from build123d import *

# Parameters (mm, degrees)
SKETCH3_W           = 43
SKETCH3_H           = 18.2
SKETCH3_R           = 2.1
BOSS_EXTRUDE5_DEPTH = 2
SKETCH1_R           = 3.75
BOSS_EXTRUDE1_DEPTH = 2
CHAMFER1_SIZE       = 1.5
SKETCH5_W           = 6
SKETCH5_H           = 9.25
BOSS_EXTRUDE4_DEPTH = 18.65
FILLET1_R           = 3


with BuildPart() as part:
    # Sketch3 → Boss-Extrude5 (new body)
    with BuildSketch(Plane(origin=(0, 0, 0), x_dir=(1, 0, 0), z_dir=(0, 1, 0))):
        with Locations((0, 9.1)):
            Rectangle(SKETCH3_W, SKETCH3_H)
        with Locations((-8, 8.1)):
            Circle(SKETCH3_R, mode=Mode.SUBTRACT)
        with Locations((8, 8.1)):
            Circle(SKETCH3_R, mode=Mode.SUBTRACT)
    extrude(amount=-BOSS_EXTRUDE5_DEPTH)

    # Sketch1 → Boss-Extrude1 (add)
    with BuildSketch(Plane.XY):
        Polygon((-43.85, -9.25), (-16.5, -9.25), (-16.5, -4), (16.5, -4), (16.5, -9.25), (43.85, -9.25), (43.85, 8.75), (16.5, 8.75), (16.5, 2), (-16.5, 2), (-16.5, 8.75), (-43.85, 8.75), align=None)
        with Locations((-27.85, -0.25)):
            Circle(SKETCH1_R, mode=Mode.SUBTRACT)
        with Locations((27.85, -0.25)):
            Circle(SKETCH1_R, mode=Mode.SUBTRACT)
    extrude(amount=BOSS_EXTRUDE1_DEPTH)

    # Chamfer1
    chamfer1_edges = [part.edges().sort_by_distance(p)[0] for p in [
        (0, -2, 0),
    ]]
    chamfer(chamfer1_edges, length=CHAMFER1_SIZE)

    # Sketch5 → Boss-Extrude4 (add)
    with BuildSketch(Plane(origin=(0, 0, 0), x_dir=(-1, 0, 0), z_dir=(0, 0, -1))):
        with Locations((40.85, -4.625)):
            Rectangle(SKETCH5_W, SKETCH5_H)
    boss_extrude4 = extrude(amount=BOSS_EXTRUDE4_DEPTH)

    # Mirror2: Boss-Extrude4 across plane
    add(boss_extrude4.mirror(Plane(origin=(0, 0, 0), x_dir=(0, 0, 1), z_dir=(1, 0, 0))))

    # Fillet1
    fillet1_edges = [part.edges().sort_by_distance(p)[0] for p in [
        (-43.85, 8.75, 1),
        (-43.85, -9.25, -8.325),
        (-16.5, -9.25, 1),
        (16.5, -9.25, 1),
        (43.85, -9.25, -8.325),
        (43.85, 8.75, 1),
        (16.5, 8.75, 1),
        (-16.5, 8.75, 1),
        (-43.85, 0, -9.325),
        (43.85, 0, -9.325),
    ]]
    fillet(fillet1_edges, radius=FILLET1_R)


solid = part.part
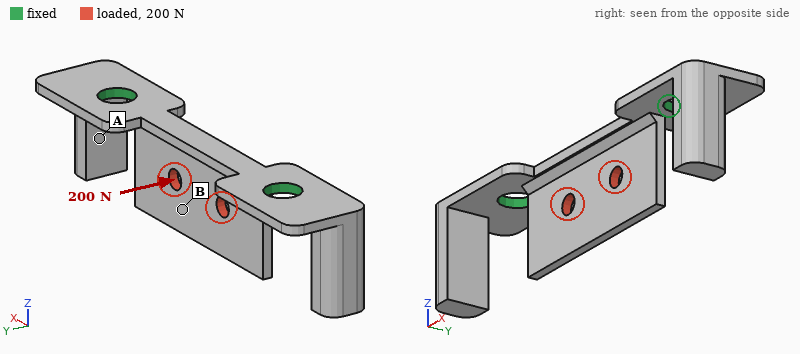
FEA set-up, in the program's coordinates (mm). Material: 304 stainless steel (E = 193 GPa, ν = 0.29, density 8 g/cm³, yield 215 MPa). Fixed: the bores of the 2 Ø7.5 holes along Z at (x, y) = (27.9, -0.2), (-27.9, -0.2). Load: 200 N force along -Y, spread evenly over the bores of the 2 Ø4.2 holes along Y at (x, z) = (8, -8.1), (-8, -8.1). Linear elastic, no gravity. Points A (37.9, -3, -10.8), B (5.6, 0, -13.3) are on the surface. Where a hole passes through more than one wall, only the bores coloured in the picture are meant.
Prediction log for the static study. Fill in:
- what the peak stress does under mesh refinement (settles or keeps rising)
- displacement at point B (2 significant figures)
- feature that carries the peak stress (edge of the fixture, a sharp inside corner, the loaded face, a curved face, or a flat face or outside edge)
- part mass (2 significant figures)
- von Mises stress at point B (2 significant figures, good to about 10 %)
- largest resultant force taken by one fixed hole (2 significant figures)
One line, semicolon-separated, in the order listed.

keeps rising; 59 µm; a sharp inside corner; 45 g; 26 MPa; 100 N
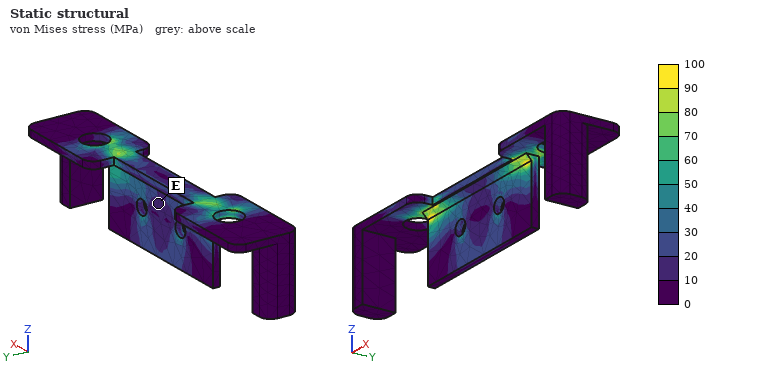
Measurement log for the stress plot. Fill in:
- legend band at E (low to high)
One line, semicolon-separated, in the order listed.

10 to 20 MPa
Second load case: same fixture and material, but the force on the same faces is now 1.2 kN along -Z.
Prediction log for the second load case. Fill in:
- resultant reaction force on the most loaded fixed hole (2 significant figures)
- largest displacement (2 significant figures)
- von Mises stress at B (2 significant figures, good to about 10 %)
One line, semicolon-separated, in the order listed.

760 N; 15 µm; 33 MPa
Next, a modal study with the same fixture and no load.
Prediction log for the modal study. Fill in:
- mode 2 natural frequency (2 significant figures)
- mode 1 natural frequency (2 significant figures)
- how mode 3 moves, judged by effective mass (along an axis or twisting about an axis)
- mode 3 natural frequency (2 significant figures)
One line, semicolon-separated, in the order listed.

2100 Hz; 2100 Hz; along Y; 2800 Hz
